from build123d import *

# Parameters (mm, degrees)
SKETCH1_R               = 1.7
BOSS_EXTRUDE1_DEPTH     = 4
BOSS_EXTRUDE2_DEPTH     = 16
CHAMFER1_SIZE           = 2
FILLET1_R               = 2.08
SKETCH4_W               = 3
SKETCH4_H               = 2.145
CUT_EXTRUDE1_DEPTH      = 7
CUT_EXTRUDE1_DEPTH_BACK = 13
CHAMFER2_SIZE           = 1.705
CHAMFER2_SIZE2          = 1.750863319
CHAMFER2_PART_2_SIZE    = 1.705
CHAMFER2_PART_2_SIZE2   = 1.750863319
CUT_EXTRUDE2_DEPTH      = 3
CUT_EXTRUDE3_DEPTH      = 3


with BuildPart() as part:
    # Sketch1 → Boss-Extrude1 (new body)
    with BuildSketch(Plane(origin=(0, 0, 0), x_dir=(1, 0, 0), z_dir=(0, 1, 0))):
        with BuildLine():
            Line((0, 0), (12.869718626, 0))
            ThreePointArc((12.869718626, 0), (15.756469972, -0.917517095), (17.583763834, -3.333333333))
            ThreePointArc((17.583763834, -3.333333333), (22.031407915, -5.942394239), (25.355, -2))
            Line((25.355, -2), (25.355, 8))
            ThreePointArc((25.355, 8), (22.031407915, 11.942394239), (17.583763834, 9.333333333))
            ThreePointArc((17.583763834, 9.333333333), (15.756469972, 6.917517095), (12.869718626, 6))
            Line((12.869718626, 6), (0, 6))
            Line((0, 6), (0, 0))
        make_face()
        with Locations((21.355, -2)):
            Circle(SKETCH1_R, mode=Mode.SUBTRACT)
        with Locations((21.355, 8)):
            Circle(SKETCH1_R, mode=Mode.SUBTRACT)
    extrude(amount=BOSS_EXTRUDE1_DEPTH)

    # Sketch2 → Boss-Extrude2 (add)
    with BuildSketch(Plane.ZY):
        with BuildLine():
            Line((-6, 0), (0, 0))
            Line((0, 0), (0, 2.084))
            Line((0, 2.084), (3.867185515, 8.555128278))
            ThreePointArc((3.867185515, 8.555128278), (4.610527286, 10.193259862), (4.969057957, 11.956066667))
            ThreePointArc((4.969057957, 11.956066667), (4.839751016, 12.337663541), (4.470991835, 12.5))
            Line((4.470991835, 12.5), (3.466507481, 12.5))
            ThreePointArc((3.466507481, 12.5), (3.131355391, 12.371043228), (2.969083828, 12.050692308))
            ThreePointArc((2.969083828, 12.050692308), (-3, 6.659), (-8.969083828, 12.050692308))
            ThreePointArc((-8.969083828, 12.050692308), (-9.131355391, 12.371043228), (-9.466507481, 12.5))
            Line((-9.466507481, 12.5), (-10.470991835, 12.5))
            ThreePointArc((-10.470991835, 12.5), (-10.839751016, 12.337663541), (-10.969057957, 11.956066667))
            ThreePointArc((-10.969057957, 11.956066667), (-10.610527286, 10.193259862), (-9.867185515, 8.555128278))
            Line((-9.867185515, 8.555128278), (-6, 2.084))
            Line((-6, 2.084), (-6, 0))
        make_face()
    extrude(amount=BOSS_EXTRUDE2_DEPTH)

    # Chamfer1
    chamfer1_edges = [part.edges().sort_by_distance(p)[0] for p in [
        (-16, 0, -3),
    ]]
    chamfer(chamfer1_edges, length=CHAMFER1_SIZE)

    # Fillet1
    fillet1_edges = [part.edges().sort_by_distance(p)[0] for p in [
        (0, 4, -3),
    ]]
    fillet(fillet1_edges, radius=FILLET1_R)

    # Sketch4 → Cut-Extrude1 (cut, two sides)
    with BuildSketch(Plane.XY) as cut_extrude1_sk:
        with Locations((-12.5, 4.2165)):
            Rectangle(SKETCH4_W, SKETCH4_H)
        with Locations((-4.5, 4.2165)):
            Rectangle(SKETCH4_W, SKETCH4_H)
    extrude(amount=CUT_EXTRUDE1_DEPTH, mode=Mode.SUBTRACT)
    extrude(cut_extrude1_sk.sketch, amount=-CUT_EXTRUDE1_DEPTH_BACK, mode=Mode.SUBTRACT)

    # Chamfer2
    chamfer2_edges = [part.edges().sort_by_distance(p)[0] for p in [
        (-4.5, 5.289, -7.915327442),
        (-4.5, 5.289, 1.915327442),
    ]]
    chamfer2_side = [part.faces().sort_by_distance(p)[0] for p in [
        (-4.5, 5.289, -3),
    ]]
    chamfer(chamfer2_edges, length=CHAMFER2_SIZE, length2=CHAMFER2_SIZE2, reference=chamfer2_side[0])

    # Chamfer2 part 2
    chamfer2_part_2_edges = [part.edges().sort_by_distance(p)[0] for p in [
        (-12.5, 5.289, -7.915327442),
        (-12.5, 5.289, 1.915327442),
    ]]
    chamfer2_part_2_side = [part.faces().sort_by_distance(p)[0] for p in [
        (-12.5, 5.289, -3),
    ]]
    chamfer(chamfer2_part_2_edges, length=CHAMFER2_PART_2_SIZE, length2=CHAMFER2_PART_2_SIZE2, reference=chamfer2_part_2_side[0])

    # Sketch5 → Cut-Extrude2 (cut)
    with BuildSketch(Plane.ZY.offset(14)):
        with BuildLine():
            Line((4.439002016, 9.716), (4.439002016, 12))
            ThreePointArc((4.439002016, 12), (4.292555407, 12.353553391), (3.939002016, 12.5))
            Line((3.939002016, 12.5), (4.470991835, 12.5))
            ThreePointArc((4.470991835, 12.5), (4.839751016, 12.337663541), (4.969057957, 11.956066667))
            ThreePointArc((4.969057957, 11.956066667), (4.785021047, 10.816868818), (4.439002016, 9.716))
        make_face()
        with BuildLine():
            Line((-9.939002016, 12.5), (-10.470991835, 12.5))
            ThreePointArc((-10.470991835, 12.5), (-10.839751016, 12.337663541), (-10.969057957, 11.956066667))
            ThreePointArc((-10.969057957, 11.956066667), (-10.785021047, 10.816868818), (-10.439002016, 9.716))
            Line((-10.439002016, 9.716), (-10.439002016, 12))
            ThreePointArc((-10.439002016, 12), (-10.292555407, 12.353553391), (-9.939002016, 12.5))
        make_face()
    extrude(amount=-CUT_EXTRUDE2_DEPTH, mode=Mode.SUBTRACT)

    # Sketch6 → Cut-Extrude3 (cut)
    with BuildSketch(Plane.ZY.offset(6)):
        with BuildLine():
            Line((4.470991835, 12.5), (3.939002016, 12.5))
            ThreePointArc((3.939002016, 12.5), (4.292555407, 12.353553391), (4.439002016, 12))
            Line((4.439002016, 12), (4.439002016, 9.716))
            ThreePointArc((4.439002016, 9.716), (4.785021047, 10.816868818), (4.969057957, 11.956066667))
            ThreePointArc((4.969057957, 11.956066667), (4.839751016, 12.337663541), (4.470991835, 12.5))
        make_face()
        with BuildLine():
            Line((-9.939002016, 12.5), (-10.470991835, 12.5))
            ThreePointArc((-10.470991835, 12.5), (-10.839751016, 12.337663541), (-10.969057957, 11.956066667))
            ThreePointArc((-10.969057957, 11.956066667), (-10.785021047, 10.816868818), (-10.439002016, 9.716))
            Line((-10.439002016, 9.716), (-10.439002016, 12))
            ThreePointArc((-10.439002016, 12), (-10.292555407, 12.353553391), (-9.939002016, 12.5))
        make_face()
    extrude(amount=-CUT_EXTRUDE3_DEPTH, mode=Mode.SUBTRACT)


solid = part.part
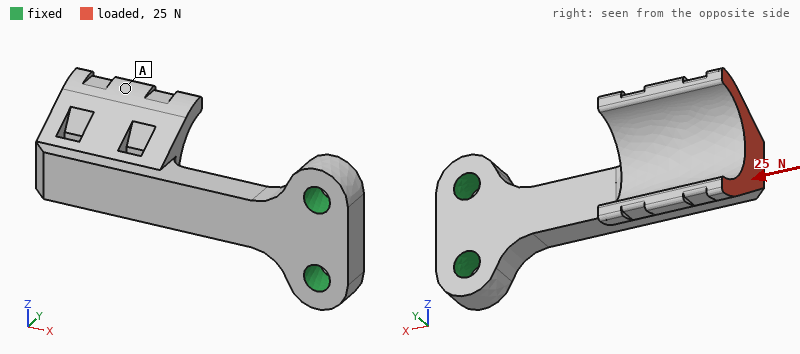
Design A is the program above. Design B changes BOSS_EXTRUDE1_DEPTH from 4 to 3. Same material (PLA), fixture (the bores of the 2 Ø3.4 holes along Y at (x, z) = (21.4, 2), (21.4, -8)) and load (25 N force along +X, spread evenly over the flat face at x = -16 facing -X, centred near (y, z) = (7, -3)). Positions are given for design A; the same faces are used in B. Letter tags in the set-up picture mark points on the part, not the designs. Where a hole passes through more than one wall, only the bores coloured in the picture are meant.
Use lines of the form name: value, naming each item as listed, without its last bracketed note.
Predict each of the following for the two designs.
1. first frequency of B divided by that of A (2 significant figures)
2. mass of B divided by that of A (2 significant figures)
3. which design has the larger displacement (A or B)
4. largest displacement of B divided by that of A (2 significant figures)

first frequency of B divided by that of A: 0.66
mass of B divided by that of A: 0.89
which design has the larger displacement: B
largest displacement of B divided by that of A: 2.6
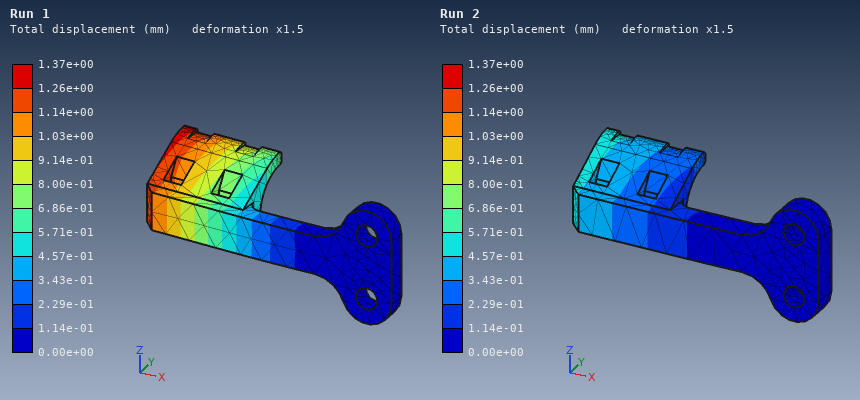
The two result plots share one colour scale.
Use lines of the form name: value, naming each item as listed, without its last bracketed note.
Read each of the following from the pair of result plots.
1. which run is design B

which run is design B: Run 1
